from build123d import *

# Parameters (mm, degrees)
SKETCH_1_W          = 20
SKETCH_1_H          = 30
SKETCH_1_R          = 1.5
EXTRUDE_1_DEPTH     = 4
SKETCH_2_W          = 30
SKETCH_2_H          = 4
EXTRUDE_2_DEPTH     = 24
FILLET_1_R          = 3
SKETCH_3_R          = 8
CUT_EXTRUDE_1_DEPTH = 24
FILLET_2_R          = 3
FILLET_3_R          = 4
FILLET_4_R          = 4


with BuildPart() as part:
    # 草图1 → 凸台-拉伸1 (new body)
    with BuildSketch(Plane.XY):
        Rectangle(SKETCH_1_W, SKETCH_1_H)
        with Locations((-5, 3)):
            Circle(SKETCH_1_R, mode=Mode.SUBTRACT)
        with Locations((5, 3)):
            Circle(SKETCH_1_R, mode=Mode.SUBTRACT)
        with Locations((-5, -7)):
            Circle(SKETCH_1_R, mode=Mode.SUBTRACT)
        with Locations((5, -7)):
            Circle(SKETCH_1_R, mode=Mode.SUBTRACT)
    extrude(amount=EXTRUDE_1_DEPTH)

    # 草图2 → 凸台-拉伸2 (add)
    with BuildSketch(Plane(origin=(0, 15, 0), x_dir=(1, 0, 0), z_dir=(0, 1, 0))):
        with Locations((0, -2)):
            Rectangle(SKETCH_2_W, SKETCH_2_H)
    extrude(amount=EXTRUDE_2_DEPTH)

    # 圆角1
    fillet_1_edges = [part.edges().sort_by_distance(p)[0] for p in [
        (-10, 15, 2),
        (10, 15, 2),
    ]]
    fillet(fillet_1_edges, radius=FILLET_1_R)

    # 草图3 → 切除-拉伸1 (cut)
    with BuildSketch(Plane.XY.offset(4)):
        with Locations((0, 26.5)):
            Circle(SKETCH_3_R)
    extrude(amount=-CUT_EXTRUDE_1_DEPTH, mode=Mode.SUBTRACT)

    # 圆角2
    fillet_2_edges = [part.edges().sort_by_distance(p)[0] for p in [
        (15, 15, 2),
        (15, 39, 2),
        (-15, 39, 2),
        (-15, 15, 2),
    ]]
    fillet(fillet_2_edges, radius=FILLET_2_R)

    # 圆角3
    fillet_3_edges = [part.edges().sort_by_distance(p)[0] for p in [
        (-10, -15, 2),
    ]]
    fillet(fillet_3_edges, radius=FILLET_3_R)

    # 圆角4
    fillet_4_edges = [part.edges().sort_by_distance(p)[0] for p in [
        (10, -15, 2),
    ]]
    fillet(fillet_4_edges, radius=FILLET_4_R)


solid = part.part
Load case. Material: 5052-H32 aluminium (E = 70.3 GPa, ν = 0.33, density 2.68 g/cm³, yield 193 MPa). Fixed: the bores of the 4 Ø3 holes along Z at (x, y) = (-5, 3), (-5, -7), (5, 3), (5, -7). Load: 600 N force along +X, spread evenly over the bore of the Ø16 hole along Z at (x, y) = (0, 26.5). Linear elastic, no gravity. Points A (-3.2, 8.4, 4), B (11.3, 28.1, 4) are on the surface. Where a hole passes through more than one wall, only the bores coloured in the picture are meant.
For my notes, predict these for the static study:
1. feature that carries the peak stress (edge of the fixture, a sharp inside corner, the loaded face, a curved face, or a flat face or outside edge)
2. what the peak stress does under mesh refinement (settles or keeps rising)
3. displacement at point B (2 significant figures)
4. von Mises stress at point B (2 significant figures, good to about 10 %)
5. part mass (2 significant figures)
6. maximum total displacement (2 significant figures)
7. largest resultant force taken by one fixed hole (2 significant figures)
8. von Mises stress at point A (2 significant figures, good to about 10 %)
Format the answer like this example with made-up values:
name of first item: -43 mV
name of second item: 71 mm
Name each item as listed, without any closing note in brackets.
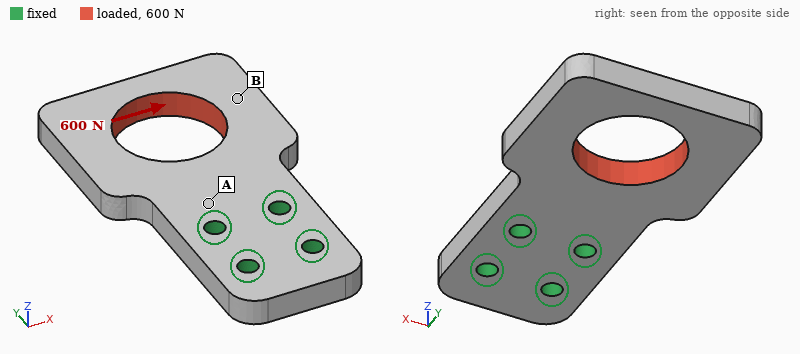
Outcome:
feature that carries the peak stress: edge of the fixture
what the peak stress does under mesh refinement: keeps rising
displacement at point B: 39 µm
von Mises stress at point B: 11 MPa
part mass: 12 g
maximum total displacement: 57 µm
largest resultant force taken by one fixed hole: 990 N
von Mises stress at point A: 27 MPa
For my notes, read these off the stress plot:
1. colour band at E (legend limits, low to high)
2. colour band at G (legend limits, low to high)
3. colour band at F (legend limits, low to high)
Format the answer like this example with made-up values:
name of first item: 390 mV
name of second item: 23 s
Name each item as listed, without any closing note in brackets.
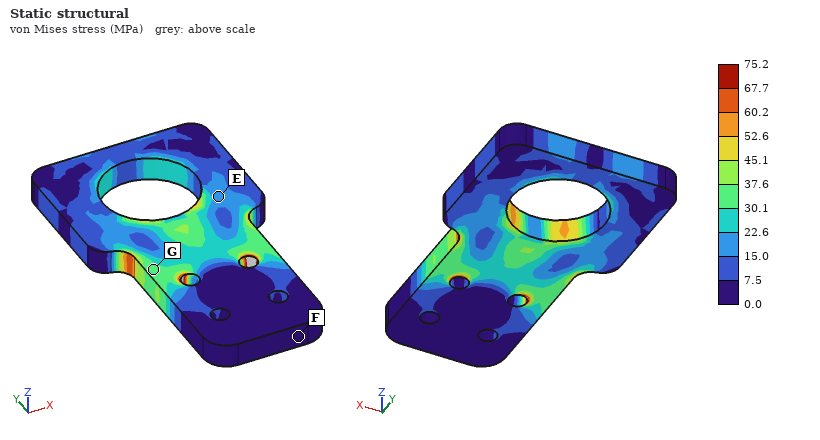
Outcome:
colour band at E: 15.0 to 22.6 MPa
colour band at G: 30.1 to 37.6 MPa
colour band at F: 0.0 to 7.5 MPa
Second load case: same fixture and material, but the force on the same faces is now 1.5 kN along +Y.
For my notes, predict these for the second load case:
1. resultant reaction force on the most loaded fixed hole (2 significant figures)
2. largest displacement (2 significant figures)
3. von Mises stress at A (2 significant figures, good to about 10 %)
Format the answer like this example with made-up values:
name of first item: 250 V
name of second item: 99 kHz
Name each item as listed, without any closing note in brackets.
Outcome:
resultant reaction force on the most loaded fixed hole: 660 N
largest displacement: 19 µm
von Mises stress at A: 14 MPa
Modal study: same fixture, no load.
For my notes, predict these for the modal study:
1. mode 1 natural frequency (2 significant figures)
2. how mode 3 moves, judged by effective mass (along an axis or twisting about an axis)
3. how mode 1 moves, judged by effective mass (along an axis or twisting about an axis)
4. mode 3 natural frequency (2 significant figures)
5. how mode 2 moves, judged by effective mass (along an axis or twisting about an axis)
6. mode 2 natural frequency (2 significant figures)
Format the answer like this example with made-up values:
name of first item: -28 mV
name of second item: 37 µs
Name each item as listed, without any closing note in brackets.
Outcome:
mode 1 natural frequency: 2400 Hz
how mode 3 moves, judged by effective mass: along X
how mode 1 moves, judged by effective mass: along Z
mode 3 natural frequency: 7700 Hz
how mode 2 moves, judged by effective mass: twisting about Y
mode 2 natural frequency: 5100 Hz
